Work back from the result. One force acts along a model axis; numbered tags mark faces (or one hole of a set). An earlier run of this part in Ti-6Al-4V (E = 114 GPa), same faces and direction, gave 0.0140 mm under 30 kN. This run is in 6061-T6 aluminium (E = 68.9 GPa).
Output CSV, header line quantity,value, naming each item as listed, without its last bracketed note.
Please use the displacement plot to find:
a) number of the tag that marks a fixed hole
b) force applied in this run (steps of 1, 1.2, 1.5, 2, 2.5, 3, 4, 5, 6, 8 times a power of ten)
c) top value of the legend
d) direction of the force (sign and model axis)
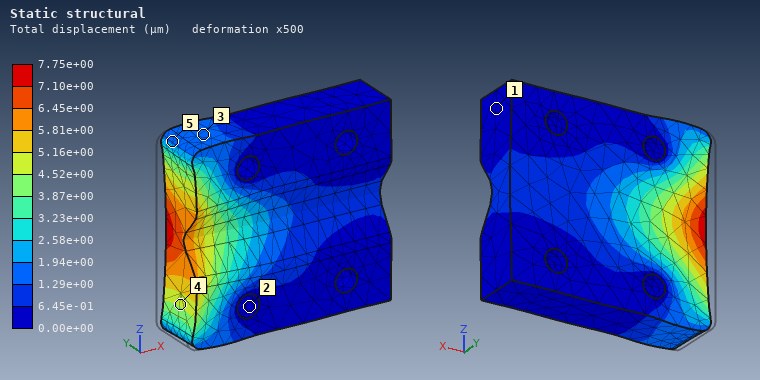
quantity,value
number of the tag that marks a fixed hole,2
force applied in this run,10 kN
top value of the legend,7.75e+00 µm
direction of the force,+X
